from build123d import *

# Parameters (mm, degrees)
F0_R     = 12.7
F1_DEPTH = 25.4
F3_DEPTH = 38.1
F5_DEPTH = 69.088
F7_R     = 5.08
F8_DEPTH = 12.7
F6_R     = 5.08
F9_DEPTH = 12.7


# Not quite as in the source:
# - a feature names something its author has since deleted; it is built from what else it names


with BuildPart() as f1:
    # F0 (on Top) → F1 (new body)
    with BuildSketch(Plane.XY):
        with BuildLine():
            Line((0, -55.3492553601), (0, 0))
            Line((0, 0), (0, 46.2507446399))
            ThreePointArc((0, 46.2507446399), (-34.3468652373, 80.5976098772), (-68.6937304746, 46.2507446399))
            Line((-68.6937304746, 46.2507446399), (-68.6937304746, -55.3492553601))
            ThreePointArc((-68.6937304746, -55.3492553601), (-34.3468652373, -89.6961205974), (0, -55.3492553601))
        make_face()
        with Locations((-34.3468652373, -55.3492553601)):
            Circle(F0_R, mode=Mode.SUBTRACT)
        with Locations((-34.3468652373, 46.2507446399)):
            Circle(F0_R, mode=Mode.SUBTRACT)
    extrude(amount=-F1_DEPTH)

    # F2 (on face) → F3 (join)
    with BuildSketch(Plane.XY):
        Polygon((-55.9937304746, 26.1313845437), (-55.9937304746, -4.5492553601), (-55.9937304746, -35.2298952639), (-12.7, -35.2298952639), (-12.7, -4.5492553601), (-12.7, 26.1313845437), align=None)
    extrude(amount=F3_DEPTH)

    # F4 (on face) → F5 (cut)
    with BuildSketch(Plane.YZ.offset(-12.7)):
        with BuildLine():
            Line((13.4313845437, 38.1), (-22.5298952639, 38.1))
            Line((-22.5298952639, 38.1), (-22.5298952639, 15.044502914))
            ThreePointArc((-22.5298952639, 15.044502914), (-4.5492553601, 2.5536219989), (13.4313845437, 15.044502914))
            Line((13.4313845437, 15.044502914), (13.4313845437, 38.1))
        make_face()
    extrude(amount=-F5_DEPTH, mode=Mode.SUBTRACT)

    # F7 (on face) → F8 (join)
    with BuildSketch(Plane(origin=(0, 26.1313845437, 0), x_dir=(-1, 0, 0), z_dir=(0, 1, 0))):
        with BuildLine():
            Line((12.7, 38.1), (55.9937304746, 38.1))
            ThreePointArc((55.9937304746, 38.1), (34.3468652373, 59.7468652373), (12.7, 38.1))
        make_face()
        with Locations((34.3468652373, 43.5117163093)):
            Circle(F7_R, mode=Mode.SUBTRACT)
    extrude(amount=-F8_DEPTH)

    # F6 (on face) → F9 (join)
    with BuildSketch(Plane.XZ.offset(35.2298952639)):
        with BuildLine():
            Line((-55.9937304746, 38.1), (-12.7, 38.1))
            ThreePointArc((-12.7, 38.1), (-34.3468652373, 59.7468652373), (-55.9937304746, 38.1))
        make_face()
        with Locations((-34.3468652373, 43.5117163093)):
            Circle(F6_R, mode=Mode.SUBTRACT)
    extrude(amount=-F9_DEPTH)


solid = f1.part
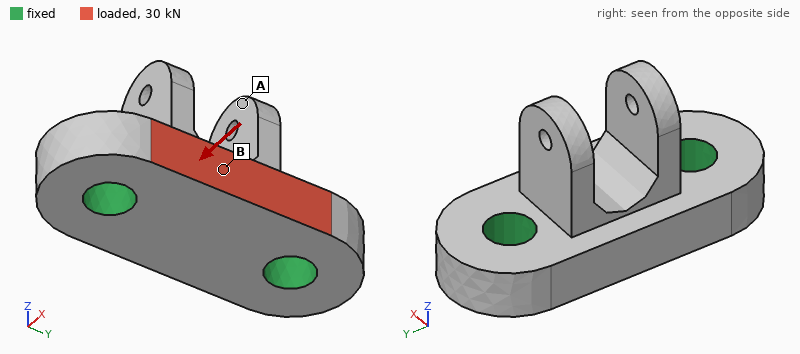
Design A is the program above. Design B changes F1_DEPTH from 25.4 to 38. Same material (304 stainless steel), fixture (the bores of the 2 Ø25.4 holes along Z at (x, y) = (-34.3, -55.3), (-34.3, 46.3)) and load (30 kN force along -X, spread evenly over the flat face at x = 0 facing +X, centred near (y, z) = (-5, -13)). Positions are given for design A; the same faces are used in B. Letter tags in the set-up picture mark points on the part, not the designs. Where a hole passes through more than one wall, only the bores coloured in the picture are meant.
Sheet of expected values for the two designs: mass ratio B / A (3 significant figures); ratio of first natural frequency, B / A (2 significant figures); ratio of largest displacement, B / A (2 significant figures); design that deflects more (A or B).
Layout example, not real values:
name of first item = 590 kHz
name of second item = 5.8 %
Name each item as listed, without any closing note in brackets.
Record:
mass ratio B / A = 1.39
ratio of first natural frequency, B / A = 1.0
ratio of largest displacement, B / A = 0.67
design that deflects more = A
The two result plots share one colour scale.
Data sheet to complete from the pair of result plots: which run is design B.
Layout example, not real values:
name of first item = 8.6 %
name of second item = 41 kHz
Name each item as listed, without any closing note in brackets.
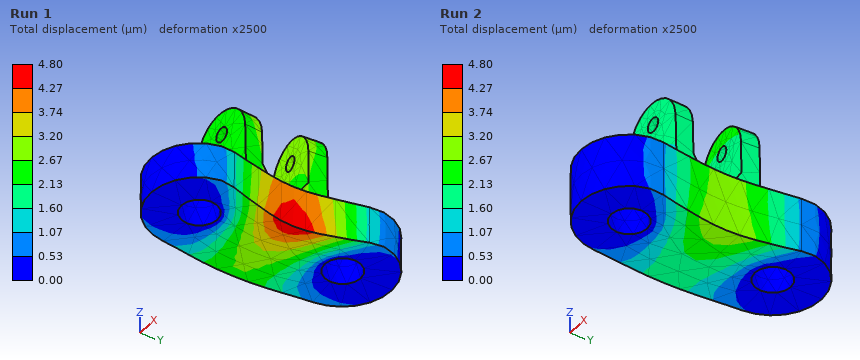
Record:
which run is design B = Run 2
